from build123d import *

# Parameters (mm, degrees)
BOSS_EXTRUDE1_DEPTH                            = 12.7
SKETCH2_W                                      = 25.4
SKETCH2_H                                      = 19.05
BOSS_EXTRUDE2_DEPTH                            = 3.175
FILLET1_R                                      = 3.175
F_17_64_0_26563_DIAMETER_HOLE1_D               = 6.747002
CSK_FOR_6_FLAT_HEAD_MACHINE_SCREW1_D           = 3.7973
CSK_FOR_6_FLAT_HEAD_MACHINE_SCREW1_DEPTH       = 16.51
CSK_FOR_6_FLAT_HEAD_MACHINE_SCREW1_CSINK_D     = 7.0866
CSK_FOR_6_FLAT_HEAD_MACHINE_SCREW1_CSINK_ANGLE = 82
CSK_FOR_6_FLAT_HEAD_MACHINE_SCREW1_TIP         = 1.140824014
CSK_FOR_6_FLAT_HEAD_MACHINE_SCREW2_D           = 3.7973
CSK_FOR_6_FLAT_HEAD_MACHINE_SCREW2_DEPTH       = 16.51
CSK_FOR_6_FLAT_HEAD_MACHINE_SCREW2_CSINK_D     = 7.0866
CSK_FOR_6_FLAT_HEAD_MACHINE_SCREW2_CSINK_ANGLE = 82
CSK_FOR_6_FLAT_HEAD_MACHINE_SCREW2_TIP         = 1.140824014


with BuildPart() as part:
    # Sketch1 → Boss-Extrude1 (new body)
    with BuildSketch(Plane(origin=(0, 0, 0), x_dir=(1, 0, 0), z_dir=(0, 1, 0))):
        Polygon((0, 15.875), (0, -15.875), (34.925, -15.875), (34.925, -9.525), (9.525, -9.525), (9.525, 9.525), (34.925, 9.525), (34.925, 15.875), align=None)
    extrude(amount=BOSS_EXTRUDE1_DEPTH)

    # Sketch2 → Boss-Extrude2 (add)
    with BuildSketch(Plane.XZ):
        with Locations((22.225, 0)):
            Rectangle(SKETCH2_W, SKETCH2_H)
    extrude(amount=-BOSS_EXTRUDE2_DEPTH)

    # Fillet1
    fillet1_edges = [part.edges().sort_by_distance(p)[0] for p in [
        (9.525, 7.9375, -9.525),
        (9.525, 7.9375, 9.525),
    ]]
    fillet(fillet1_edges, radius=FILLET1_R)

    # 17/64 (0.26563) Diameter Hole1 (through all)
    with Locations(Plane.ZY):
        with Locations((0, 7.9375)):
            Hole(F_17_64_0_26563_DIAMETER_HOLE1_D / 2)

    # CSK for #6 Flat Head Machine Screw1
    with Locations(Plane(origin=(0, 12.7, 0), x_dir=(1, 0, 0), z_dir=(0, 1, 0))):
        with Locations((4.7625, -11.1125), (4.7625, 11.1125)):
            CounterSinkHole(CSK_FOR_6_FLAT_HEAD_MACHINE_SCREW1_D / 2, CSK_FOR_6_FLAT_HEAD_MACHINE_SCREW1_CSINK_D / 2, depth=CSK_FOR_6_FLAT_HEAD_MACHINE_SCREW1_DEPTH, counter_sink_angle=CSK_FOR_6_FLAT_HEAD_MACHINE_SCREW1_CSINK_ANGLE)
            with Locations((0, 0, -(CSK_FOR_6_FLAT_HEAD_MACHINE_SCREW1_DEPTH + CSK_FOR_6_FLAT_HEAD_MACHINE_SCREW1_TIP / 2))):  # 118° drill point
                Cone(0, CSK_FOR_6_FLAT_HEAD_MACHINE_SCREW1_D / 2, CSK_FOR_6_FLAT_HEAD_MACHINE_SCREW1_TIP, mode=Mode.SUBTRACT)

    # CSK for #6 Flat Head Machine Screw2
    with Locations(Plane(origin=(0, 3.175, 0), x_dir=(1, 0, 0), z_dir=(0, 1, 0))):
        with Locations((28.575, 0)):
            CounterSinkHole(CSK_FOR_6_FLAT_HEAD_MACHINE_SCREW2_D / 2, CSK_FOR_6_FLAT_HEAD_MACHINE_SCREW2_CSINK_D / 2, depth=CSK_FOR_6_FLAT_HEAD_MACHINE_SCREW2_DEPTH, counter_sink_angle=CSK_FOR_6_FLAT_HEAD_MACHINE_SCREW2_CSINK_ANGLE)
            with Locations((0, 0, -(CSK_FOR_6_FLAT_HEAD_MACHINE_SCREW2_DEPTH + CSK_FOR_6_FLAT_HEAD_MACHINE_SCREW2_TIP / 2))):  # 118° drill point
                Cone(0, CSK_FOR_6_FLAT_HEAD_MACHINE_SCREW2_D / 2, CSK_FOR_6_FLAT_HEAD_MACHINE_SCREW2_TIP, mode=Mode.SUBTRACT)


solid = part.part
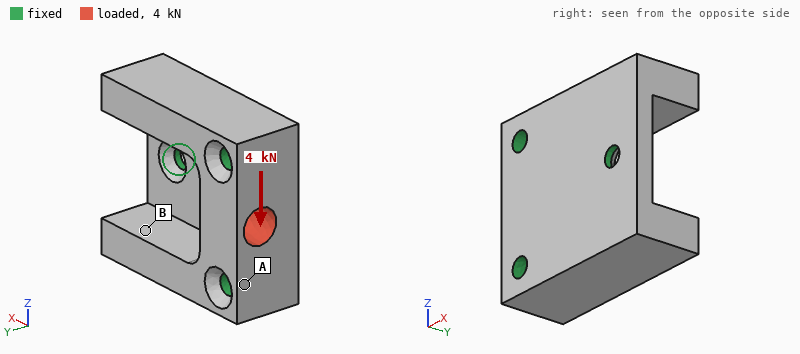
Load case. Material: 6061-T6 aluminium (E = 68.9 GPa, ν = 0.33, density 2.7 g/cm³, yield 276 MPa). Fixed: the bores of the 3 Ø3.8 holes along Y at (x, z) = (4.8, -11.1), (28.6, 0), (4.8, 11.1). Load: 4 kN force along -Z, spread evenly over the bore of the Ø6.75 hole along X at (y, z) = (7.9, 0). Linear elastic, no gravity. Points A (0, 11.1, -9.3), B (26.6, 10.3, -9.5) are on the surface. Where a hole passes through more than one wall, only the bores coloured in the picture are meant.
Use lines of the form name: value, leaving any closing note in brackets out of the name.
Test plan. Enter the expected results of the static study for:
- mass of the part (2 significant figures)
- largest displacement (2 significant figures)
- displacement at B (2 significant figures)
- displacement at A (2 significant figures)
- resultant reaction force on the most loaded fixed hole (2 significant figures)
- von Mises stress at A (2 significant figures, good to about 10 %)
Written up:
mass of the part: 24 g
largest displacement: 4.2 µm
displacement at B: 0.89 µm
displacement at A: 1.5 µm
resultant reaction force on the most loaded fixed hole: 2.0 kN
von Mises stress at A: 12 MPa
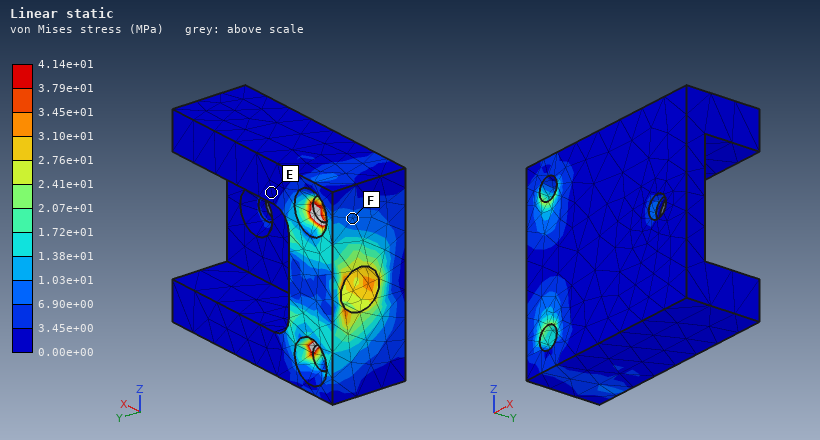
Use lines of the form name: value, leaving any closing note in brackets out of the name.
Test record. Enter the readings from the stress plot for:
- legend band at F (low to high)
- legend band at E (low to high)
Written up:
legend band at F: 6.90e+00 to 1.03e+01 MPa
legend band at E: 0.00e+00 to 3.45e+00 MPa
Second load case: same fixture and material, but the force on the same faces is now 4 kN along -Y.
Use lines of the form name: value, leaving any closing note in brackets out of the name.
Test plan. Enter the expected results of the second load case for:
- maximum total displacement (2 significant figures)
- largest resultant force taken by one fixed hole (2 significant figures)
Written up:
maximum total displacement: 13 µm
largest resultant force taken by one fixed hole: 2.0 kN
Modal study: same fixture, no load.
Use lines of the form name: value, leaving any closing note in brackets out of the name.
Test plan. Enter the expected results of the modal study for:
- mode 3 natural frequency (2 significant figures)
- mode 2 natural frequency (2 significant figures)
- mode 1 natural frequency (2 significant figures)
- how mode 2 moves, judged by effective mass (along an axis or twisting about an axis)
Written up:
mode 3 natural frequency: 22 kHz
mode 2 natural frequency: 13 kHz
mode 1 natural frequency: 12 kHz
how mode 2 moves, judged by effective mass: along Y
